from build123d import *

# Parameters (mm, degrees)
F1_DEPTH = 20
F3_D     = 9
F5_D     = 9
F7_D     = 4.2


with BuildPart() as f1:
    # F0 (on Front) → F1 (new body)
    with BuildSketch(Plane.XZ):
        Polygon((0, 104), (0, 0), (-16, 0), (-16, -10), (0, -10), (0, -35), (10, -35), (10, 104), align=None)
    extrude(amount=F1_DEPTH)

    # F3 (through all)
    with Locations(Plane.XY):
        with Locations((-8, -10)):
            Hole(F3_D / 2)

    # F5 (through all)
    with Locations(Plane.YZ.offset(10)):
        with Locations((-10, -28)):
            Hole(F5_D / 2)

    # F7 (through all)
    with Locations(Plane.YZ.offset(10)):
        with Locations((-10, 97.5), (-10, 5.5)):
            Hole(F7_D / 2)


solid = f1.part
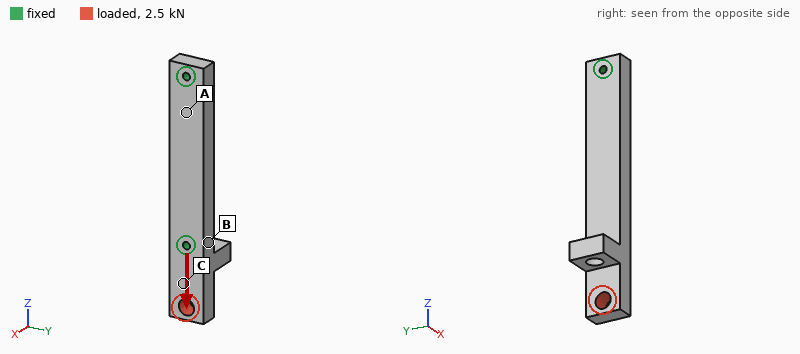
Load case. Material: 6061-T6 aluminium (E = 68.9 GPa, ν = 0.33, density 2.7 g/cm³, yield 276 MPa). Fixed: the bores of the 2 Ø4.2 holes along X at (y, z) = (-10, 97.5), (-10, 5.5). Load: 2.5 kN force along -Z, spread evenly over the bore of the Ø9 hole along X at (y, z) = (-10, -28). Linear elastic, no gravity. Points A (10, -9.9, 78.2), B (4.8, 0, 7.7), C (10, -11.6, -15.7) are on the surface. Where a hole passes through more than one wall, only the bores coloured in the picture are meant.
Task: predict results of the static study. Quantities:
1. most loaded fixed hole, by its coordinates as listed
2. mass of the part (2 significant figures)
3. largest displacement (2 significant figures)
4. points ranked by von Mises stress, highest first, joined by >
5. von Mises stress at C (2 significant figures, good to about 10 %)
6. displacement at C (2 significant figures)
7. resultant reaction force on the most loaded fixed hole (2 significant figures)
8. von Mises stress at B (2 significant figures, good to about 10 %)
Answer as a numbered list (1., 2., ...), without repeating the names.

1. (-10, 5.5)
2. 80 g
3. 13 µm
4. C > B > A
5. 11 MPa
6. 4.8 µm
7. 2.4 kN
8. 6.2 MPa
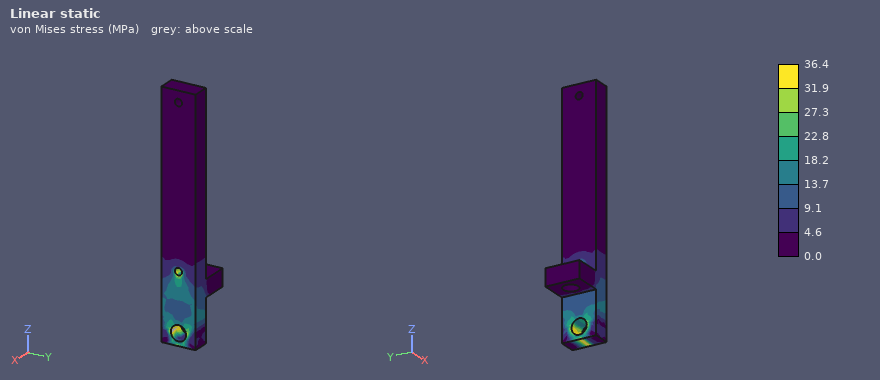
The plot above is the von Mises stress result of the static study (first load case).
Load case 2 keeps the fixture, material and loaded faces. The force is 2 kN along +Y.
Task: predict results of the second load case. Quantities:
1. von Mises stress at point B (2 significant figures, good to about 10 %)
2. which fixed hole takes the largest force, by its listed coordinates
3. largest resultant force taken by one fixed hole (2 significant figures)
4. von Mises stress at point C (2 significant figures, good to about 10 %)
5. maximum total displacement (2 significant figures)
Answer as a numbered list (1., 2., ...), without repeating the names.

1. 66 MPa
2. (-10, 5.5)
3. 2.4 kN
4. 29 MPa
5. 0.18 mm
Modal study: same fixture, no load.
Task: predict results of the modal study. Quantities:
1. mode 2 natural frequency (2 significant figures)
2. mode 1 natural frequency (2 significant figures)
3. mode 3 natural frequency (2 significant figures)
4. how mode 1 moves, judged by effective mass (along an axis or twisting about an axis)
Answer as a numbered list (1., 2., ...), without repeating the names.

1. 5500 Hz
2. 4800 Hz
3. 5600 Hz
4. twisting about Y
